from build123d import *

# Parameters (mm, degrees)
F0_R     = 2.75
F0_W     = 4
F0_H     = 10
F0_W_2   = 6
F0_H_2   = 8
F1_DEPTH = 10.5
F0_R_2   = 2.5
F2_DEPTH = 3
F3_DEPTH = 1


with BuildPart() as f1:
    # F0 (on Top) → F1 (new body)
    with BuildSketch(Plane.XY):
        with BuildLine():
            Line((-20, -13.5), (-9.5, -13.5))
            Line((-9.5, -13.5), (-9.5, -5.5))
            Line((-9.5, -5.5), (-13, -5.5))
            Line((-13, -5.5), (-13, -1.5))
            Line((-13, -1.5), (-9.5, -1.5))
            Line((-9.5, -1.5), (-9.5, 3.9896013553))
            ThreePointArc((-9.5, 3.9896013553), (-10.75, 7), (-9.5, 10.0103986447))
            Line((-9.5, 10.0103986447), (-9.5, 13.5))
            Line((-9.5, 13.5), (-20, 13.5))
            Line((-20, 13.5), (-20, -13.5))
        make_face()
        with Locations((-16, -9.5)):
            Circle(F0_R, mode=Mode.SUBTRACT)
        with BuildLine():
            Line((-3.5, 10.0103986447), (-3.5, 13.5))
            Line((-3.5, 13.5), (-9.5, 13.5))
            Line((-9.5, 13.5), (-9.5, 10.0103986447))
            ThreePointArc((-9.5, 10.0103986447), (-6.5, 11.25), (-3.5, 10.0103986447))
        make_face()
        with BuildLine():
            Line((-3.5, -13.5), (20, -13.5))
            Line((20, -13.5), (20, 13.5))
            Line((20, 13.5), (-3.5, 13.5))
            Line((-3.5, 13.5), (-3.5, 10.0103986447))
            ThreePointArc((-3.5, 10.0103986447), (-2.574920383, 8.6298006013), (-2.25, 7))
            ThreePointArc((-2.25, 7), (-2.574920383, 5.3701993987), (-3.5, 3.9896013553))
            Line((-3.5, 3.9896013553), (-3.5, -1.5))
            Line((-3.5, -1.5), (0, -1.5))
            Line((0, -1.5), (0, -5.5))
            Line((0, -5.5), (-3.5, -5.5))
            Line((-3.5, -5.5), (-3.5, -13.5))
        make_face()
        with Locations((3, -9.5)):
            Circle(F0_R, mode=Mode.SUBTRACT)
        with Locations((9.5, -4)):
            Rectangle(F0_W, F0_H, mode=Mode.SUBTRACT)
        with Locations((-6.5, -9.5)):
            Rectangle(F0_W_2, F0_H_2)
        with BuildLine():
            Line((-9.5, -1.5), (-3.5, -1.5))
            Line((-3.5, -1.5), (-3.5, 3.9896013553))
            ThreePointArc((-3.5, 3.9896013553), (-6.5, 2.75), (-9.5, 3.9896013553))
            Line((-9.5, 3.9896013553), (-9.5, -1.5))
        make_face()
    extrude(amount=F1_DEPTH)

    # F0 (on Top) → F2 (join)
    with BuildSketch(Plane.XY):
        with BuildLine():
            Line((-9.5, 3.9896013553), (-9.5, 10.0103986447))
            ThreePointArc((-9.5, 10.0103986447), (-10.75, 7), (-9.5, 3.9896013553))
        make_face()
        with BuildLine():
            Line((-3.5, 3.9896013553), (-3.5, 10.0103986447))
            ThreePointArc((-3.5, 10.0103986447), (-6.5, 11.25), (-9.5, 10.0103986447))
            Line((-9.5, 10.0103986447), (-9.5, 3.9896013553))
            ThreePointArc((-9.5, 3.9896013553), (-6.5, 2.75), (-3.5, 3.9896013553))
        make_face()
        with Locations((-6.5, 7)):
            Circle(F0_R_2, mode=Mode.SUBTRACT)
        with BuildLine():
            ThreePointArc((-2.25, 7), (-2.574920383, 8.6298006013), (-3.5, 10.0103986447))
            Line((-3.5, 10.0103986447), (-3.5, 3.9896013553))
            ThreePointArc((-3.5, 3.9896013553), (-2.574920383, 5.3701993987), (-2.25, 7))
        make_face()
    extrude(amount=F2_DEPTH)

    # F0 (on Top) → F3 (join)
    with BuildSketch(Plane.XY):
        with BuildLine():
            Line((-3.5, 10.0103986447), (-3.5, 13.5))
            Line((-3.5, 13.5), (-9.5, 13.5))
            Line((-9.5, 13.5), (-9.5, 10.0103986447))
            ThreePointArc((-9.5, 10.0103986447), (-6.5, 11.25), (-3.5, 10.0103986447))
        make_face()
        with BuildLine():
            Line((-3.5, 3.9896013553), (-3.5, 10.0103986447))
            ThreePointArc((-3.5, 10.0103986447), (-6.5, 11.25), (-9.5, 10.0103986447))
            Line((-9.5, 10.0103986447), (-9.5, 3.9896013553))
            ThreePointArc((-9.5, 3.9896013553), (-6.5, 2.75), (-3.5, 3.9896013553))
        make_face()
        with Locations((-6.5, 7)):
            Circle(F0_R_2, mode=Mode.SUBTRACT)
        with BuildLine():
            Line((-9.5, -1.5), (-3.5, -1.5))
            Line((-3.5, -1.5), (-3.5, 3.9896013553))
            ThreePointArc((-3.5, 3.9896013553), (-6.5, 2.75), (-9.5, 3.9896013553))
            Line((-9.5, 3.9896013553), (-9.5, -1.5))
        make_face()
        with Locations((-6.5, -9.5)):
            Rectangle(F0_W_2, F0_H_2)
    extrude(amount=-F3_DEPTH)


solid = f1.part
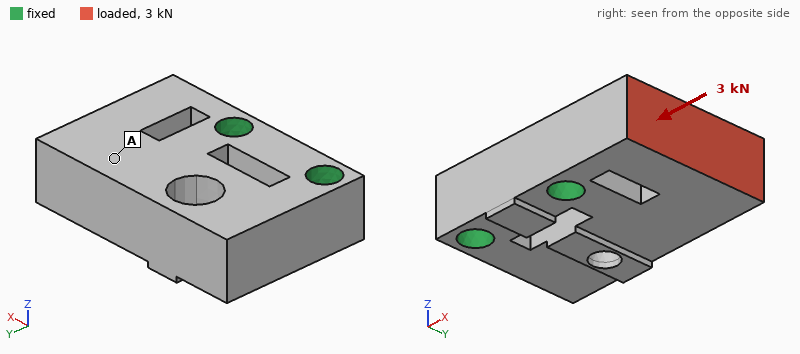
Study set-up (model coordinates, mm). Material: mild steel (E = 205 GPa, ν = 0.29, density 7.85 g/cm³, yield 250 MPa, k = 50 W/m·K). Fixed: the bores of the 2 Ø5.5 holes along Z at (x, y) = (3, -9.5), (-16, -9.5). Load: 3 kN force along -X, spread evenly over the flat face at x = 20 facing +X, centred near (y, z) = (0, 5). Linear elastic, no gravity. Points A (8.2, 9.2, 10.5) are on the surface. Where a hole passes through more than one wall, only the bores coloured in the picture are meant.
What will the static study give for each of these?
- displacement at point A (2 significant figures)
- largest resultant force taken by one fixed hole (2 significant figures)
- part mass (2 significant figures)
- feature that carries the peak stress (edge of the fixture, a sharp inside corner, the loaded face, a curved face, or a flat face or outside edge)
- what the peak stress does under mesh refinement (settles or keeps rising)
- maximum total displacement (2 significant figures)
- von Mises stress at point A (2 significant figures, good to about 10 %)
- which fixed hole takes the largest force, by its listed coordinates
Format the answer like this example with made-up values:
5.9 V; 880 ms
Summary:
5.5 µm; 2.3 kN; 75 g; edge of the fixture; keeps rising; 7.5 µm; 8.8 MPa; (3, -9.5)
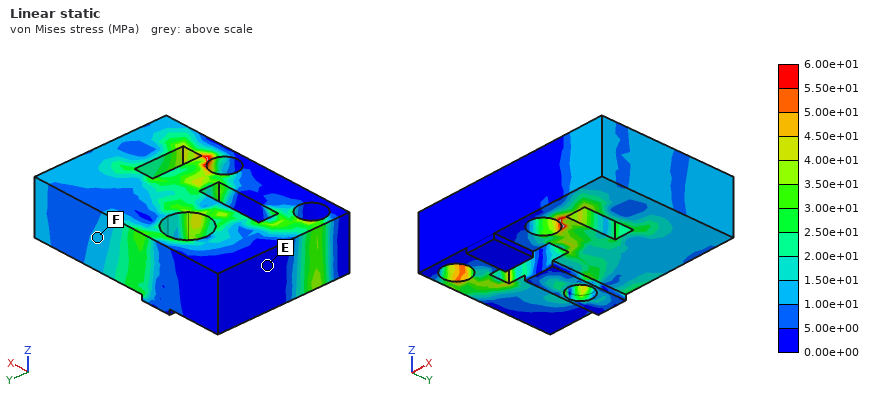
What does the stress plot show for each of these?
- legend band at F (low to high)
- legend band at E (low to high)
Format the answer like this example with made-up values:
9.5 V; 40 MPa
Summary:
1.00e+01 to 1.50e+01 MPa; 0.00e+00 to 5.00e+00 MPa
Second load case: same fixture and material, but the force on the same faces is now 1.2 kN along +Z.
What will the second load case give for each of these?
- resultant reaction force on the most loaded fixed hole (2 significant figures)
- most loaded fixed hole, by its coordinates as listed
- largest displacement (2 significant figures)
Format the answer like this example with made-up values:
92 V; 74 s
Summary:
1.5 kN; (3, -9.5); 21 µm
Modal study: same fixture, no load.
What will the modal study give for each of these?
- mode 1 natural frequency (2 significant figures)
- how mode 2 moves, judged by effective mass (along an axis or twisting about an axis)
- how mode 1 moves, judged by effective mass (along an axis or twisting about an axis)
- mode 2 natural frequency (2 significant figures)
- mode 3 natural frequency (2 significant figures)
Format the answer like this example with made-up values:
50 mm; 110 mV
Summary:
9800 Hz; along X; along Z; 14 kHz; 16 kHz
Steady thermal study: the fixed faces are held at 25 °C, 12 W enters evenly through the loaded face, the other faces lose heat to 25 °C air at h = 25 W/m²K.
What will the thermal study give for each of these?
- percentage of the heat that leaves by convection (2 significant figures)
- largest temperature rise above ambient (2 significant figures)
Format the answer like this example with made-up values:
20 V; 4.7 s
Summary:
6.9 %; 26 K
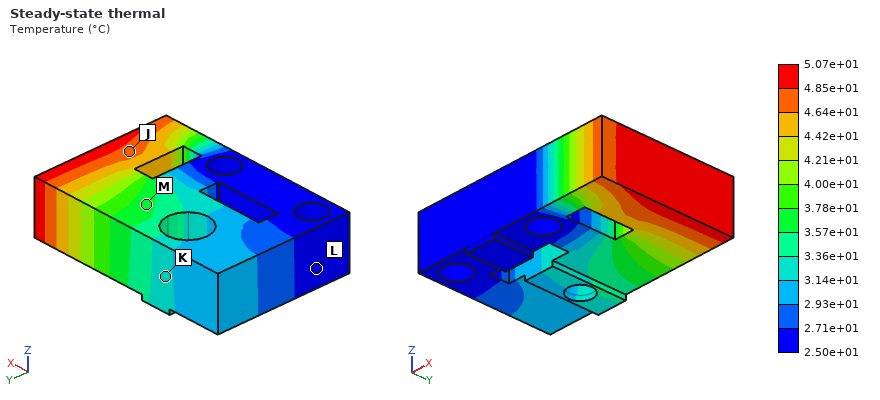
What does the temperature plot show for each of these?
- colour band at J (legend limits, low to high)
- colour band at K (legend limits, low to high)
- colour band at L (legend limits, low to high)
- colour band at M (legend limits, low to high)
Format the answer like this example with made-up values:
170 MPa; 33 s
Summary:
4.64e+01 to 4.85e+01 °C; 3.14e+01 to 3.36e+01 °C; 2.50e+01 to 2.71e+01 °C; 3.57e+01 to 3.78e+01 °C
